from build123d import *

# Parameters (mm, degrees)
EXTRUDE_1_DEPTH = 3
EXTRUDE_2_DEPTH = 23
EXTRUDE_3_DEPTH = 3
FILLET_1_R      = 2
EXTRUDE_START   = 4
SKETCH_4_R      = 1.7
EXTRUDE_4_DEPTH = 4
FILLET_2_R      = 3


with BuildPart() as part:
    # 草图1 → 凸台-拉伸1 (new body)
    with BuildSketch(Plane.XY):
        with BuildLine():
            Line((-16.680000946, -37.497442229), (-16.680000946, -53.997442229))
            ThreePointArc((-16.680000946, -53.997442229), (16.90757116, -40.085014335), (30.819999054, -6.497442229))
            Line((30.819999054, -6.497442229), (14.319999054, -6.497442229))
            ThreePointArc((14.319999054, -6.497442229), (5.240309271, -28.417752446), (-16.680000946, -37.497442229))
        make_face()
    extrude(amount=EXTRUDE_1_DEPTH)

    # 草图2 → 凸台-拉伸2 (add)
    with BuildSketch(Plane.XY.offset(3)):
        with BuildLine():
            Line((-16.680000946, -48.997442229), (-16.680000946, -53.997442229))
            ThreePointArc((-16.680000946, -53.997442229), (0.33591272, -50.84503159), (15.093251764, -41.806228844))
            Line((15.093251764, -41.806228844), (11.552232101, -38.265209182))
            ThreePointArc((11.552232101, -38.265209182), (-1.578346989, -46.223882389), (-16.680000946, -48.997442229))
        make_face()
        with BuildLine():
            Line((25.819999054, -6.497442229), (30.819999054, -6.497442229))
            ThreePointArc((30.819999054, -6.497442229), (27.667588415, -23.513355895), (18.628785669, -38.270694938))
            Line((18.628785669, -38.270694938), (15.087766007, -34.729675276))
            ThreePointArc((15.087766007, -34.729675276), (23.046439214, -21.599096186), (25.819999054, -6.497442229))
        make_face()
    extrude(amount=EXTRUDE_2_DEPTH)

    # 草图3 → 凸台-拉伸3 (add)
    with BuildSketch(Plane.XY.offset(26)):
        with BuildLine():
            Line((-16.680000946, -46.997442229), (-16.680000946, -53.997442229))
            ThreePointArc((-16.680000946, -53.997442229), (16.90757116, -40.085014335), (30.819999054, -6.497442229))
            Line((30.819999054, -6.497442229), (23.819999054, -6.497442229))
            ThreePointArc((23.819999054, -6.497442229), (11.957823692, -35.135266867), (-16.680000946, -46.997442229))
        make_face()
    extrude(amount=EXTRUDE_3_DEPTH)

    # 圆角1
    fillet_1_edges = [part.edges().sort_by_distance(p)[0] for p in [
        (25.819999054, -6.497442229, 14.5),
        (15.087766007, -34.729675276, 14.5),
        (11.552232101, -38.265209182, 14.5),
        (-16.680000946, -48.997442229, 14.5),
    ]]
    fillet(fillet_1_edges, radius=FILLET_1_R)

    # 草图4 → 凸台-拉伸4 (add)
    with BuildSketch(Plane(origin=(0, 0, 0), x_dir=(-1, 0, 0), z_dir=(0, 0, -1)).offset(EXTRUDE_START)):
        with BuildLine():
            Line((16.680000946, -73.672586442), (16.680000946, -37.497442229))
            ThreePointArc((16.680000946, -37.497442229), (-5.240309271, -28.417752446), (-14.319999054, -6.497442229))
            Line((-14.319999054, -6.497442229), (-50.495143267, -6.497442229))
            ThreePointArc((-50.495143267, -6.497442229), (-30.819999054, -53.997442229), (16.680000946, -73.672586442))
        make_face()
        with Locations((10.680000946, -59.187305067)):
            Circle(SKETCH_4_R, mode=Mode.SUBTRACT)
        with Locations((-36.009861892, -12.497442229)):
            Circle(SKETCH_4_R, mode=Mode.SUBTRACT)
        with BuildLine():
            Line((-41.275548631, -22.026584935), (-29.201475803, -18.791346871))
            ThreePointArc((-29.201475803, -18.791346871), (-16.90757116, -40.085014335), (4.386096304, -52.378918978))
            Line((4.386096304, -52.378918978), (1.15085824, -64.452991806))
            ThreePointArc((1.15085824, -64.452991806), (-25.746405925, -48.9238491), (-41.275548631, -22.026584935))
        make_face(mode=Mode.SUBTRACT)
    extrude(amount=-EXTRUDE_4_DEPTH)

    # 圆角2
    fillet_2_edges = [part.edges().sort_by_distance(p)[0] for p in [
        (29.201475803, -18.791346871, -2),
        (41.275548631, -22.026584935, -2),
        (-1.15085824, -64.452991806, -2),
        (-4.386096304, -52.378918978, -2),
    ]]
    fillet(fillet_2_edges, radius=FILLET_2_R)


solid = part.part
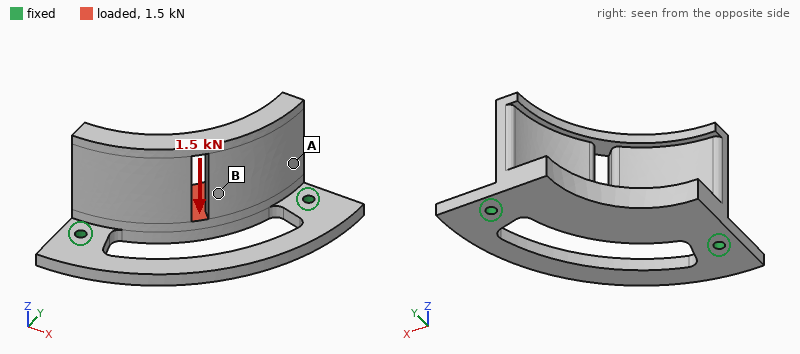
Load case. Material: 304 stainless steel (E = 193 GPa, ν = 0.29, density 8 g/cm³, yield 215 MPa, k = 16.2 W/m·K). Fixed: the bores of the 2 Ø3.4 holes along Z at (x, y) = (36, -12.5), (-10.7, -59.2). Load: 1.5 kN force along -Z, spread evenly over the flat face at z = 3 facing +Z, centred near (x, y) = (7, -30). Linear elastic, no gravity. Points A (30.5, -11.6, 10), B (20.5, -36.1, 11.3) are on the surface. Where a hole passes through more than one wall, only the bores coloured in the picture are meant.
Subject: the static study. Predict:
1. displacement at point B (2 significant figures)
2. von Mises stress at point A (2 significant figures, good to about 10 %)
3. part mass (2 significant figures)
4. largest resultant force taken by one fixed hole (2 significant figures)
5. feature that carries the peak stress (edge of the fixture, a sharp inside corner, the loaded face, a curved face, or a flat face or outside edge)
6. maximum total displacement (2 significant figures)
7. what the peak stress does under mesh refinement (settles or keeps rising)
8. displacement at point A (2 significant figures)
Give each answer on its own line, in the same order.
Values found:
18 µm
24 MPa
160 g
850 N
edge of the fixture
44 µm
keeps rising
20 µm
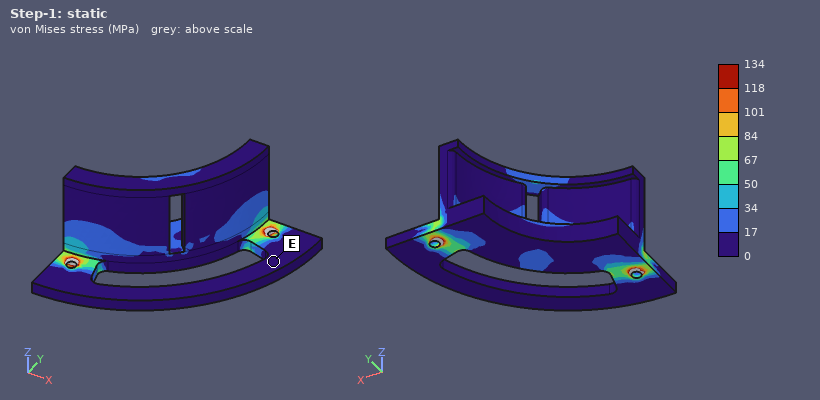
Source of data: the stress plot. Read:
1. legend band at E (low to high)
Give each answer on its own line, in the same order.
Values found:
0 to 17 MPa
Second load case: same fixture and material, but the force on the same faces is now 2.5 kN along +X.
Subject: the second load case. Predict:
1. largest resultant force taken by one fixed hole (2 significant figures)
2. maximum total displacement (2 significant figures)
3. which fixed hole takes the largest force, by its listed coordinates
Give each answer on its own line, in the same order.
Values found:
1.6 kN
61 µm
(36, -12.5)
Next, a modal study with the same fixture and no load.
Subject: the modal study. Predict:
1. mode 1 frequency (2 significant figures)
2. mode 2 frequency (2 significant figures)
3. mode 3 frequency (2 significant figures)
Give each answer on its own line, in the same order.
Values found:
1900 Hz
2700 Hz
4700 Hz
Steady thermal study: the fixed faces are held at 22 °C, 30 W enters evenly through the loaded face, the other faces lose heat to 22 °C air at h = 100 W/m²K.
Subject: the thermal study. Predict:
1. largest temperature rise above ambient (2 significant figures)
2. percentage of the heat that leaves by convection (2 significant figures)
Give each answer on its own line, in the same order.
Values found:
79 K
77 %
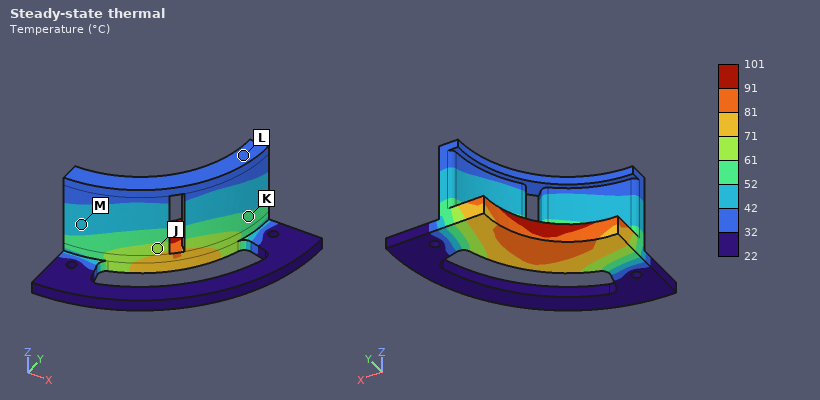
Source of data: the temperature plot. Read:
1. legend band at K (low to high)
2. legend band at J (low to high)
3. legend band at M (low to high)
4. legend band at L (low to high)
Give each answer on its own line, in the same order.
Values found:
52 to 61 °C
61 to 71 °C
42 to 52 °C
32 to 42 °C
